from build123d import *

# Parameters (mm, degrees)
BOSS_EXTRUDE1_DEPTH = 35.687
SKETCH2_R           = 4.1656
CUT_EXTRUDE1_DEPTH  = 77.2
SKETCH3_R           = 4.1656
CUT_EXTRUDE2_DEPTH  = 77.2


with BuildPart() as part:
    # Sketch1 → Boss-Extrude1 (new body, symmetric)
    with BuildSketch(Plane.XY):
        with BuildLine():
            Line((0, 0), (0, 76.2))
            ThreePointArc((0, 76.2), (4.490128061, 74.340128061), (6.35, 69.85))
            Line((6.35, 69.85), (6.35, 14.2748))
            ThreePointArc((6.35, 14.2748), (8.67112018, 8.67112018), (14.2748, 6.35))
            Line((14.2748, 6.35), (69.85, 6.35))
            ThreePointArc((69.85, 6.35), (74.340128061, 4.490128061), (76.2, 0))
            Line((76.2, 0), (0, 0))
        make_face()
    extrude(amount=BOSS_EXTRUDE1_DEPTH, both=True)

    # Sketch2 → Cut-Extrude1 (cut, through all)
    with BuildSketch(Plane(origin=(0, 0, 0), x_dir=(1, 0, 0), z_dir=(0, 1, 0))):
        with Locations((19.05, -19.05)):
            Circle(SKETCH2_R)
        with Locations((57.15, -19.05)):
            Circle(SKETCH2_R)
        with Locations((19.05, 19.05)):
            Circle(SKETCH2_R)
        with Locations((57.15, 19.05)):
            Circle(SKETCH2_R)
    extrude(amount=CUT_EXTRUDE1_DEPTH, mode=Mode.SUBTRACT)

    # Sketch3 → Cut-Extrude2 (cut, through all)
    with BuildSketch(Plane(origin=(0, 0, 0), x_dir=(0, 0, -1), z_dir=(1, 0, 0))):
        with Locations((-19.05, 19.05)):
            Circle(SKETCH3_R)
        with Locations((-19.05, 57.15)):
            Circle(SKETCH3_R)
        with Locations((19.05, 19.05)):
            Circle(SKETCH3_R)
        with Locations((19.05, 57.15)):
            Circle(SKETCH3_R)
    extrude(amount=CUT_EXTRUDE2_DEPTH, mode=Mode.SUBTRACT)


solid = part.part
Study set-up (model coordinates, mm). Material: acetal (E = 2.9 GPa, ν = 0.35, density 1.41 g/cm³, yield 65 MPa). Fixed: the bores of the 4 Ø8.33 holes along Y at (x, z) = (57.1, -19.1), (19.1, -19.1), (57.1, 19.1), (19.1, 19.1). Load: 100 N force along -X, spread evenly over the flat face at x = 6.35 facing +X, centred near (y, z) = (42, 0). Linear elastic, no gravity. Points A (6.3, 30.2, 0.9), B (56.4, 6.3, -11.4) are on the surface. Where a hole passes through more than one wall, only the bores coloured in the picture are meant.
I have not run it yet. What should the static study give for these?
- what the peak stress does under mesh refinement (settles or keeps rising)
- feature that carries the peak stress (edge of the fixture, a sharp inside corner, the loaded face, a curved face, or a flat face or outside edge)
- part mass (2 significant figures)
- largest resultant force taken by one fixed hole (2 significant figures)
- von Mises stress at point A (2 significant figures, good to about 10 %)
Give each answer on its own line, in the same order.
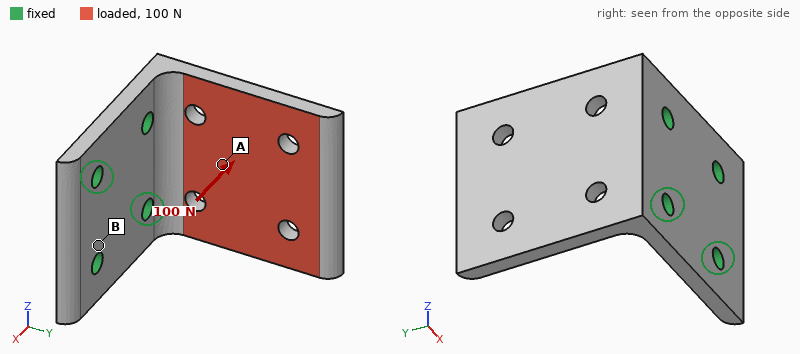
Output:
keeps rising
edge of the fixture
89 g
47 N
3.0 MPa
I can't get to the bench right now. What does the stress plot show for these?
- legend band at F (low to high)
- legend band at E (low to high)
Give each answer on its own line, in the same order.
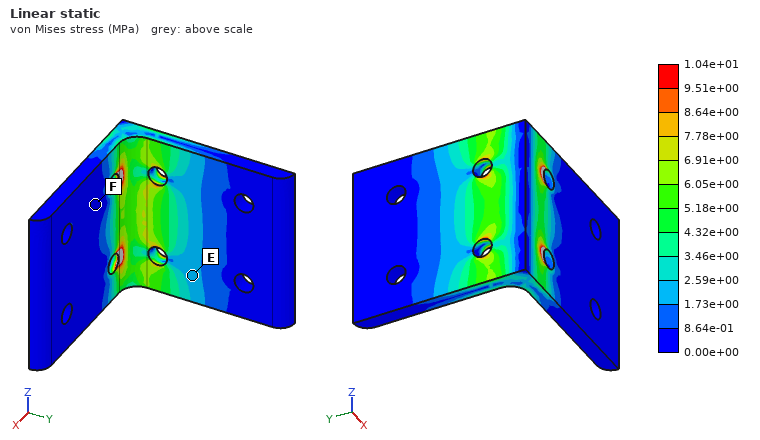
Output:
0.00e+00 to 8.64e-01 MPa
1.73e+00 to 2.59e+00 MPa
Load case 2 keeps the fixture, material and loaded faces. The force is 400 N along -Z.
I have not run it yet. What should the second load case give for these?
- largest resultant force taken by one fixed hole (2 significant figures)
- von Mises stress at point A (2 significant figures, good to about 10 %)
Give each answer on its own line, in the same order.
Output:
420 N
3.9 MPa
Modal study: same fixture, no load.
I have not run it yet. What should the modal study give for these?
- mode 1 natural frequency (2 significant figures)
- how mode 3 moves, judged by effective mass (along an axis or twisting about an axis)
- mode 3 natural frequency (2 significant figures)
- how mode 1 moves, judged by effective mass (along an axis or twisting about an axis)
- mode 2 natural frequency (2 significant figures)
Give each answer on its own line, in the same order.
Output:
250 Hz
along Z
920 Hz
along X
620 Hz
